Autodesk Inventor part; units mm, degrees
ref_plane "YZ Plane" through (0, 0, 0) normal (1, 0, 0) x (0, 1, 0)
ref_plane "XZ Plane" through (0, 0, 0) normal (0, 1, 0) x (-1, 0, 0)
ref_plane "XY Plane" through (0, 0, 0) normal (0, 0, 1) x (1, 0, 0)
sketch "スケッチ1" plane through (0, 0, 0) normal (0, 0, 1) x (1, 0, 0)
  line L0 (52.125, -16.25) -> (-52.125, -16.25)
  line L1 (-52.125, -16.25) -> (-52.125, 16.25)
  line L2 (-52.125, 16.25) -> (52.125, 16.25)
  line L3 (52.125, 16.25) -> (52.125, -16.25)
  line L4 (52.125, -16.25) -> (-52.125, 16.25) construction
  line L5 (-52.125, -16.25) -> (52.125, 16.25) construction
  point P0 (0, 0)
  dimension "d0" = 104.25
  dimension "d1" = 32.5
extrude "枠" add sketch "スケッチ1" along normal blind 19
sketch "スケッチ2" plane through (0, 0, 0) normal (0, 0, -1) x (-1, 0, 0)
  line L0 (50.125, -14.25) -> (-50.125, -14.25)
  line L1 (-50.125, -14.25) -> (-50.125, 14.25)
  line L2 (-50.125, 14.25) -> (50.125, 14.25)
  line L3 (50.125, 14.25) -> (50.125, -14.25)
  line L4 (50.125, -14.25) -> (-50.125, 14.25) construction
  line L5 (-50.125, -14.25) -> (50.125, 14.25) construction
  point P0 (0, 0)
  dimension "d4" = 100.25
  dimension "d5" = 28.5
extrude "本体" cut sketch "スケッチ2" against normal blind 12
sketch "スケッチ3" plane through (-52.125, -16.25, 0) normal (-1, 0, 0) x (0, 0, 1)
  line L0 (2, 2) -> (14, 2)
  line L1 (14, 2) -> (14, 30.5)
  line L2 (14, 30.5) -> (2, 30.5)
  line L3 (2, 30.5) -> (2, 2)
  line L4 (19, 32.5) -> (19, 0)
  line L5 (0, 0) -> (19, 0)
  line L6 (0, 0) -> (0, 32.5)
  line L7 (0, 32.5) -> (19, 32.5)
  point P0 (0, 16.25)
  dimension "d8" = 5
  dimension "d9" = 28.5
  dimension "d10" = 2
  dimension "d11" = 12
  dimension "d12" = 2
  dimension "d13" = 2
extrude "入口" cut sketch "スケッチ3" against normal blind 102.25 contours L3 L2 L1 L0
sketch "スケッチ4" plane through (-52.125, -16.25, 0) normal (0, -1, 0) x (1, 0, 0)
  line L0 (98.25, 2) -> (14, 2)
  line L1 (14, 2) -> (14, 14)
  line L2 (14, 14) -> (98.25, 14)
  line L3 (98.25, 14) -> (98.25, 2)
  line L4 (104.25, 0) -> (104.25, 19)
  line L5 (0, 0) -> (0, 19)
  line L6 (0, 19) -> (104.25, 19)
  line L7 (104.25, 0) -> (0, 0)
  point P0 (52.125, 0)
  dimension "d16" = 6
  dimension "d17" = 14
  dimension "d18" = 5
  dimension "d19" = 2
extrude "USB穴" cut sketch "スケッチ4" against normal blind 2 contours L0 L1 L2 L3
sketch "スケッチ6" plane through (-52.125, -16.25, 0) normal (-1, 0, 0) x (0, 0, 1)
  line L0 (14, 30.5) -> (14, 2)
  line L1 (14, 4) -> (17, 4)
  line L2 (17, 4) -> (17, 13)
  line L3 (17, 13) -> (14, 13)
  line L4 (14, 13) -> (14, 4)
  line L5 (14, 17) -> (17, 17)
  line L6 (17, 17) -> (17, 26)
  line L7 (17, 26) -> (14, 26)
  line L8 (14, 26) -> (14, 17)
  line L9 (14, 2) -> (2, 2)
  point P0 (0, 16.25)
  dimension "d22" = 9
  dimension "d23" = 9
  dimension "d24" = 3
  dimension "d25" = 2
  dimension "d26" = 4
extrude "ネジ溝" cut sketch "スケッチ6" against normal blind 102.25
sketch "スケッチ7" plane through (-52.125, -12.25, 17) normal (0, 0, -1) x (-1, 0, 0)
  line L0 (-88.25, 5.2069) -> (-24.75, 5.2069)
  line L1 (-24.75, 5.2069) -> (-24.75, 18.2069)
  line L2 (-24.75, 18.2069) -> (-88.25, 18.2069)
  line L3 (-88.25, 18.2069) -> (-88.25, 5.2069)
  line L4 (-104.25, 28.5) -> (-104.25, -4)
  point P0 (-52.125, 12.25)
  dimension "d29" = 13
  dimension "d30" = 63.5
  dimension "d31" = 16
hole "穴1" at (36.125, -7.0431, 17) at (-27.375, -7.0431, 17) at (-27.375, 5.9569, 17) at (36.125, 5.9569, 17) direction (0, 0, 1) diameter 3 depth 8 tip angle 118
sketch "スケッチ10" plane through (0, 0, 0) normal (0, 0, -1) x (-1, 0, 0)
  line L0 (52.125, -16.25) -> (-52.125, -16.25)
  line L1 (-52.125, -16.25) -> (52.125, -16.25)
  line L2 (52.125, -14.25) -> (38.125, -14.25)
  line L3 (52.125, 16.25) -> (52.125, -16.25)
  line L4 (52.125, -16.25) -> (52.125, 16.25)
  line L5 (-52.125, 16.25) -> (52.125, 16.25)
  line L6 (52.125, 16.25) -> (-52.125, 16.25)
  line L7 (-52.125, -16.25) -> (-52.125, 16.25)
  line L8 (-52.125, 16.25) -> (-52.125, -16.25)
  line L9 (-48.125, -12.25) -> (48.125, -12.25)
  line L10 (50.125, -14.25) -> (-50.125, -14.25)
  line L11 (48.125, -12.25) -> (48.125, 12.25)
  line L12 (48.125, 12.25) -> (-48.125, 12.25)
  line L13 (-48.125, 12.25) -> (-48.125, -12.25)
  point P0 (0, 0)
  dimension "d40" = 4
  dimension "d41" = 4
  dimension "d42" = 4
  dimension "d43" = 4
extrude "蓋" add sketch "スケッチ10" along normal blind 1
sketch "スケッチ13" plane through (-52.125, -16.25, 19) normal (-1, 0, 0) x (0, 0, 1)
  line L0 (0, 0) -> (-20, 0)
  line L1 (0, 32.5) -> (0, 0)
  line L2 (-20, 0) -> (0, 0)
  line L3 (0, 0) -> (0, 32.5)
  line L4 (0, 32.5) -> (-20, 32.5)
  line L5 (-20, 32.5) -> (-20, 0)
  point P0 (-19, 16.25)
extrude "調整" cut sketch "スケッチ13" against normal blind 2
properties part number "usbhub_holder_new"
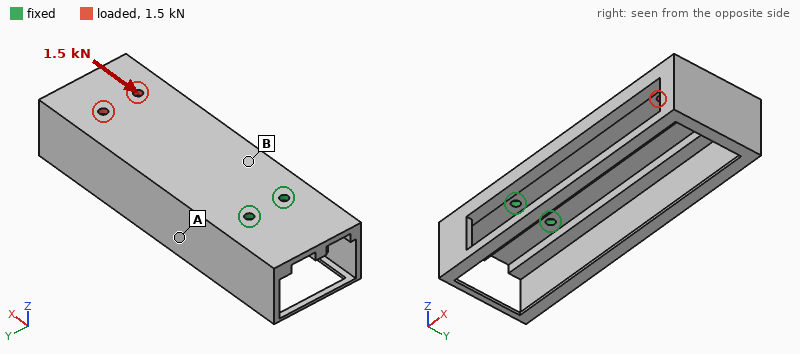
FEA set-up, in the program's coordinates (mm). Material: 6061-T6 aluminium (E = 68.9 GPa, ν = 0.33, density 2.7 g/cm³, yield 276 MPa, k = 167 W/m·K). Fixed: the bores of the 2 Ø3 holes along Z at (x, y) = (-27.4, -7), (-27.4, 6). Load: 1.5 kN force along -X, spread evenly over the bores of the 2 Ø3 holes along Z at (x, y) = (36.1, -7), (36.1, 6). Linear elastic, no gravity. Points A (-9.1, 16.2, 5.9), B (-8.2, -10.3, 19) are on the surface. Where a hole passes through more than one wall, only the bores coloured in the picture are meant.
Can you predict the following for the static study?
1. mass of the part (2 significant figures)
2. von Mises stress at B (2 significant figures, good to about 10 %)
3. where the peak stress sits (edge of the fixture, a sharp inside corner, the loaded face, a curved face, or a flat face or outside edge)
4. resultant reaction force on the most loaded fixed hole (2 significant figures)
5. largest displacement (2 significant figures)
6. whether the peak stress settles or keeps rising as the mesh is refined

45 g
21 MPa
edge of the fixture
750 N
86 µm
keeps rising
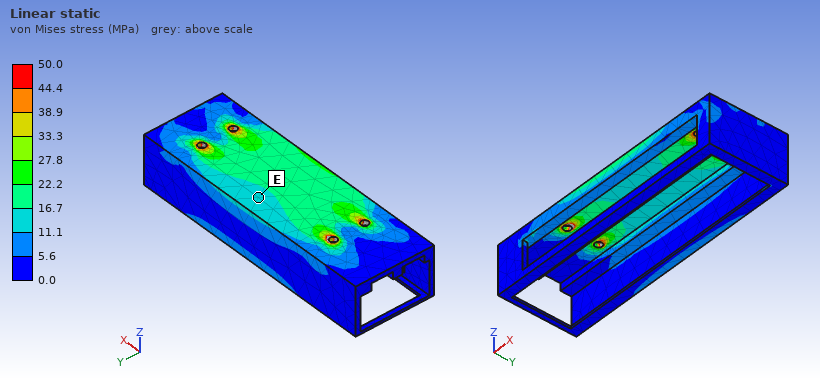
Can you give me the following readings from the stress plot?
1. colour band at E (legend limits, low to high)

11.1 to 16.7 MPa
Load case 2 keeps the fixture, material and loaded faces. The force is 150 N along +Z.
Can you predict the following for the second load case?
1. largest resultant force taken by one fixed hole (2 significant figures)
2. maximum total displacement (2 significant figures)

84 N
1.1 mm
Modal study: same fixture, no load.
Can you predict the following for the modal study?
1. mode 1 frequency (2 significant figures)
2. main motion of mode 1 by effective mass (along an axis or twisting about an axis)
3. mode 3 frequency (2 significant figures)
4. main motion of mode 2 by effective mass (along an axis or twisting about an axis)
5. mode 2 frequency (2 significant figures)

460 Hz
along Z
1500 Hz
along Y
1100 Hz
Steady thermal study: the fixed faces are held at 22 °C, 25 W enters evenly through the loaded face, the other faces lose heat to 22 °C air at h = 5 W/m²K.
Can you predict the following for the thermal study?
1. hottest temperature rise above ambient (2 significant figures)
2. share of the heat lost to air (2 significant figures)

78 K
11 %
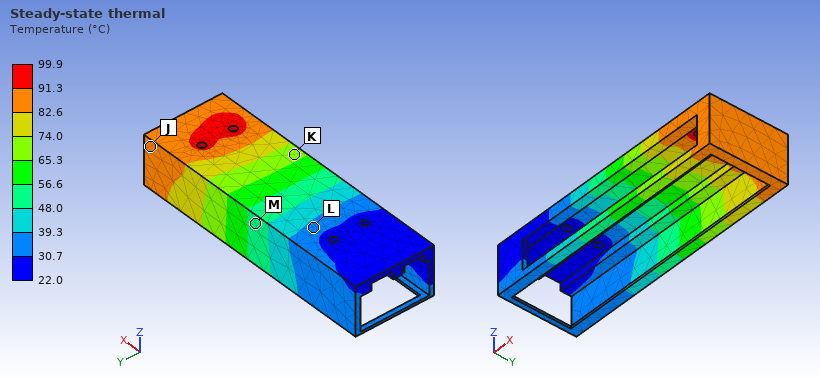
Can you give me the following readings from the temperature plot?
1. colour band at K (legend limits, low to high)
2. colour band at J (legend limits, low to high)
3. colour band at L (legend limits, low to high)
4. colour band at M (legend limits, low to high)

65.3 to 74.0 °C
82.6 to 91.3 °C
30.7 to 39.3 °C
48.0 to 56.6 °C
